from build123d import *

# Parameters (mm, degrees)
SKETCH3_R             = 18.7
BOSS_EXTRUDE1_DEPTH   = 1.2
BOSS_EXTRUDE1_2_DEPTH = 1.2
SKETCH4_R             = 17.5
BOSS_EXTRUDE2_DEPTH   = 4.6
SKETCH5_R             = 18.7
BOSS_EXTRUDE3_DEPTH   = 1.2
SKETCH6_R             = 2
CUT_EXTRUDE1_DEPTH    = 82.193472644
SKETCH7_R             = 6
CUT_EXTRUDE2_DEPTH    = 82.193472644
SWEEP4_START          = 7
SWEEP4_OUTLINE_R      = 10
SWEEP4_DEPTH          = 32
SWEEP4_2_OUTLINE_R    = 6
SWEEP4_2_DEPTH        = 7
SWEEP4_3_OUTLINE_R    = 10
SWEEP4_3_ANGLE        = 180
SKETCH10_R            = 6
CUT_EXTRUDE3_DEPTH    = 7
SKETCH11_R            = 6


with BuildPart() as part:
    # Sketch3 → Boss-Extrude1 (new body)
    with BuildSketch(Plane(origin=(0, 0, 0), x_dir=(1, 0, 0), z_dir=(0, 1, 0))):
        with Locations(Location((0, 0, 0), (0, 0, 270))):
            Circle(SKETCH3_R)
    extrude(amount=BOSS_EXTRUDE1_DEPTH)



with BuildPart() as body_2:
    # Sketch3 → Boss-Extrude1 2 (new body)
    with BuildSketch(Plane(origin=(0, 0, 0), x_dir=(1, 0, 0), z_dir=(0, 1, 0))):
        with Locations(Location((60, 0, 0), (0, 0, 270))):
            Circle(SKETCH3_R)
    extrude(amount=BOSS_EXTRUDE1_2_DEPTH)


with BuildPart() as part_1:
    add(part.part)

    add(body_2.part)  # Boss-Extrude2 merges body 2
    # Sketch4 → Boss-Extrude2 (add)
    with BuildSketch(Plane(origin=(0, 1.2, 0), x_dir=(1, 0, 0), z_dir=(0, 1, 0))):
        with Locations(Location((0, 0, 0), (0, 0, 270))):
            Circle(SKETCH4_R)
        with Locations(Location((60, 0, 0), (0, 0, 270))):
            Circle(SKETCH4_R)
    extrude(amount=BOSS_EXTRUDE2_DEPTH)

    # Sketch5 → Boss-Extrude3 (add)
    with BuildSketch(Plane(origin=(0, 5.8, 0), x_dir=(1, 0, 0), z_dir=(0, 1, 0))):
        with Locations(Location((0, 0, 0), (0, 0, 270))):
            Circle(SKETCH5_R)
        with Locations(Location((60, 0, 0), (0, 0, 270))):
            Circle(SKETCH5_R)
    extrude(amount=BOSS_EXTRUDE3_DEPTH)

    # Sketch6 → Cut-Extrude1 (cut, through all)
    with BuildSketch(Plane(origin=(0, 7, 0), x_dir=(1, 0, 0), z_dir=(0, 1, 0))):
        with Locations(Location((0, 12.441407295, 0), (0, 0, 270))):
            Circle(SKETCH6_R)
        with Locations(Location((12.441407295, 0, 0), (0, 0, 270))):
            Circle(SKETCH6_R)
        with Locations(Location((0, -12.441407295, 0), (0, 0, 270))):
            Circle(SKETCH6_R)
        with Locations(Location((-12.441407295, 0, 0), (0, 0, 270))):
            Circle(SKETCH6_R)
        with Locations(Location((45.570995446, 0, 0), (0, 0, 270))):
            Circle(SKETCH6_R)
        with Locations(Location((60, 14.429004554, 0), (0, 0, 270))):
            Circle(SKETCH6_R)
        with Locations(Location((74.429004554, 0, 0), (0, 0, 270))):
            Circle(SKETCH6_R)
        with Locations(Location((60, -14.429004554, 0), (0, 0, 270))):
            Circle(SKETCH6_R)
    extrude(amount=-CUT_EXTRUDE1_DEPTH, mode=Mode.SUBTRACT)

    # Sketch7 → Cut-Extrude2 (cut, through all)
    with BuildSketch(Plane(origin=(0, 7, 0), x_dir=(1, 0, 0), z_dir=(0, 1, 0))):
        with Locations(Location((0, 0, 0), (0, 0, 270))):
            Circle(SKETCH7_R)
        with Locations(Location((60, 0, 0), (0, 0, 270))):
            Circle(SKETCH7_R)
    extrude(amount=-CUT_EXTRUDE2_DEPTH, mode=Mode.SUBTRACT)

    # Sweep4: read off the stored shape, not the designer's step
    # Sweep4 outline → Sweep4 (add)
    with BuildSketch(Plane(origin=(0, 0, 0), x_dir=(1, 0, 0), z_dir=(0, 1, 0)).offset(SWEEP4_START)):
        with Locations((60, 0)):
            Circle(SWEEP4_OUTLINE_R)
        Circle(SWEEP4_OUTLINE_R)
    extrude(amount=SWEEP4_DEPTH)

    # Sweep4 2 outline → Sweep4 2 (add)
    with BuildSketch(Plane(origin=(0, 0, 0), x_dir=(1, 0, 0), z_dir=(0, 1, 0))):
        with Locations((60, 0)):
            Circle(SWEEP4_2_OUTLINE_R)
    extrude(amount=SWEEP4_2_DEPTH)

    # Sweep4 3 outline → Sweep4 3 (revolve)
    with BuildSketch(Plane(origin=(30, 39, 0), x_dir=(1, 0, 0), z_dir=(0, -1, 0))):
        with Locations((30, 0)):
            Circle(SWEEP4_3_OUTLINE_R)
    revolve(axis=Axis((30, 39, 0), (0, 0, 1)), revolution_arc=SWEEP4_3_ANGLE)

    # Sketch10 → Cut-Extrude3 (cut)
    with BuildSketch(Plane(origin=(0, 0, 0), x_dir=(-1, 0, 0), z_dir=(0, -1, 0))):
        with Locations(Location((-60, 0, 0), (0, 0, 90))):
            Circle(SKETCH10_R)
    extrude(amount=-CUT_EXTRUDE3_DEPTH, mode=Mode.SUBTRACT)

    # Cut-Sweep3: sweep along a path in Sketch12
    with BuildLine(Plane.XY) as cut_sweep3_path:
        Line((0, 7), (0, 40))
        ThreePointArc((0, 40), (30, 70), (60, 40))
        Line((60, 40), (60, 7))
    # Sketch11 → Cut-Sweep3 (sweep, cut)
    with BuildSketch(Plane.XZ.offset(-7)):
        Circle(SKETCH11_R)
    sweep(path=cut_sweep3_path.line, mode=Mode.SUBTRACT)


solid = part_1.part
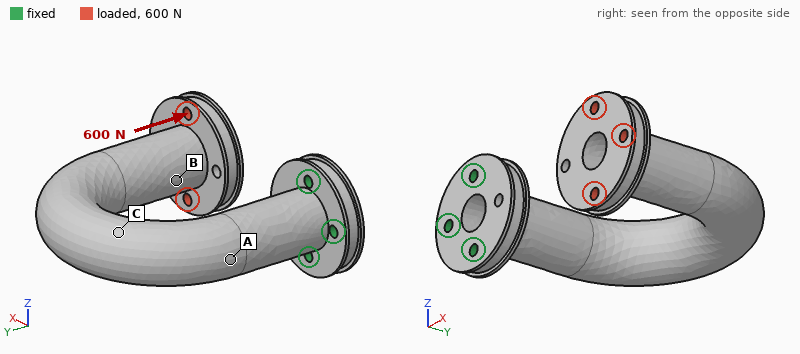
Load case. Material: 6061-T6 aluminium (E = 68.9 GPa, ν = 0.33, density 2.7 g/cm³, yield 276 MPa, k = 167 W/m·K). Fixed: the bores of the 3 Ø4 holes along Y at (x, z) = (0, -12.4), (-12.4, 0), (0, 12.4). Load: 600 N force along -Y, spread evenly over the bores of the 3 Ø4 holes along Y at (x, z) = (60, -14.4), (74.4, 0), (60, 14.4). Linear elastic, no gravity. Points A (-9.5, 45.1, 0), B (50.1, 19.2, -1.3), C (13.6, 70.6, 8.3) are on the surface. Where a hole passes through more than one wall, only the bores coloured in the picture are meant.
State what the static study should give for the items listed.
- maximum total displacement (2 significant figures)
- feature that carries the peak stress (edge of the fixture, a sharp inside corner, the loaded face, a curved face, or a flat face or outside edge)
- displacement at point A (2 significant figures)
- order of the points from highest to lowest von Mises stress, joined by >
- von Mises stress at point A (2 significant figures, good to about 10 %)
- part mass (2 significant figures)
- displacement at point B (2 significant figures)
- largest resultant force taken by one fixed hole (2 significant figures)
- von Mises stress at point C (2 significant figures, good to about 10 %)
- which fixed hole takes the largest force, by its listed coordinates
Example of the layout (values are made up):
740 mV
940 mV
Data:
0.73 mm
edge of the fixture
0.12 mm
A > C > B
46 MPa
120 g
0.41 mm
2.1 kN
30 MPa
(-12.4, 0)
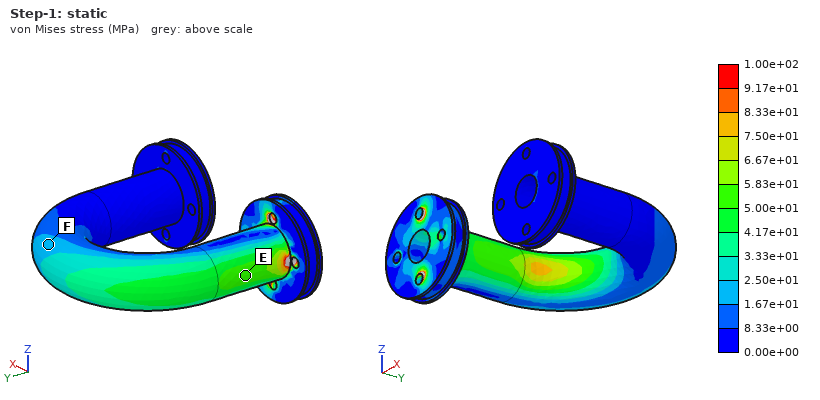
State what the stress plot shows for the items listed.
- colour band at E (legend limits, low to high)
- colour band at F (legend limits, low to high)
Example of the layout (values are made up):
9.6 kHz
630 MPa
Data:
5.00e+01 to 5.83e+01 MPa
1.67e+01 to 2.50e+01 MPa
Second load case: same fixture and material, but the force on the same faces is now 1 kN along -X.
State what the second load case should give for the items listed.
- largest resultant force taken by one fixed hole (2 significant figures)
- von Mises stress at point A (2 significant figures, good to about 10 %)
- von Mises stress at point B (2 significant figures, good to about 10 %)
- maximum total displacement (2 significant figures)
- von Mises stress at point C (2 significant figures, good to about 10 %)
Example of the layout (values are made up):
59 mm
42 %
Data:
390 N
53 MPa
20 MPa
1.2 mm
62 MPa
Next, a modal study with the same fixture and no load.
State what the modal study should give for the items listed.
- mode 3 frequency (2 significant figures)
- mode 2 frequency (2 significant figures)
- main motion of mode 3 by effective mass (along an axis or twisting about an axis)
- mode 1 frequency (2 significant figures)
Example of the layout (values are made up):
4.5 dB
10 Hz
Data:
1200 Hz
710 Hz
along X
690 Hz
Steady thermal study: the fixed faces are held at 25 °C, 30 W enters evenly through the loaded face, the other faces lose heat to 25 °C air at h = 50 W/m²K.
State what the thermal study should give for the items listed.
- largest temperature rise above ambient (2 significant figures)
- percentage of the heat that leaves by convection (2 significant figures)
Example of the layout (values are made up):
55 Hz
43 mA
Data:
58 K
80 %
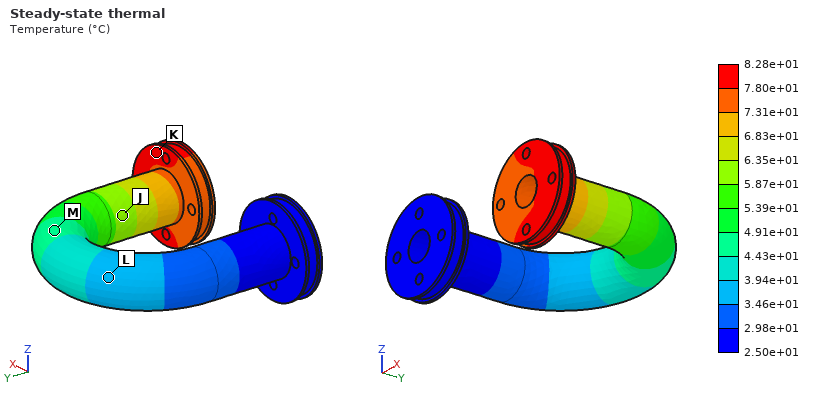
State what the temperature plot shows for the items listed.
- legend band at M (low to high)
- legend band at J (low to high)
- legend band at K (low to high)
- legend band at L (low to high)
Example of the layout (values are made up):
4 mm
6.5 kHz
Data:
4.43e+01 to 4.91e+01 °C
5.87e+01 to 6.35e+01 °C
7.80e+01 to 8.28e+01 °C
3.46e+01 to 3.94e+01 °C
